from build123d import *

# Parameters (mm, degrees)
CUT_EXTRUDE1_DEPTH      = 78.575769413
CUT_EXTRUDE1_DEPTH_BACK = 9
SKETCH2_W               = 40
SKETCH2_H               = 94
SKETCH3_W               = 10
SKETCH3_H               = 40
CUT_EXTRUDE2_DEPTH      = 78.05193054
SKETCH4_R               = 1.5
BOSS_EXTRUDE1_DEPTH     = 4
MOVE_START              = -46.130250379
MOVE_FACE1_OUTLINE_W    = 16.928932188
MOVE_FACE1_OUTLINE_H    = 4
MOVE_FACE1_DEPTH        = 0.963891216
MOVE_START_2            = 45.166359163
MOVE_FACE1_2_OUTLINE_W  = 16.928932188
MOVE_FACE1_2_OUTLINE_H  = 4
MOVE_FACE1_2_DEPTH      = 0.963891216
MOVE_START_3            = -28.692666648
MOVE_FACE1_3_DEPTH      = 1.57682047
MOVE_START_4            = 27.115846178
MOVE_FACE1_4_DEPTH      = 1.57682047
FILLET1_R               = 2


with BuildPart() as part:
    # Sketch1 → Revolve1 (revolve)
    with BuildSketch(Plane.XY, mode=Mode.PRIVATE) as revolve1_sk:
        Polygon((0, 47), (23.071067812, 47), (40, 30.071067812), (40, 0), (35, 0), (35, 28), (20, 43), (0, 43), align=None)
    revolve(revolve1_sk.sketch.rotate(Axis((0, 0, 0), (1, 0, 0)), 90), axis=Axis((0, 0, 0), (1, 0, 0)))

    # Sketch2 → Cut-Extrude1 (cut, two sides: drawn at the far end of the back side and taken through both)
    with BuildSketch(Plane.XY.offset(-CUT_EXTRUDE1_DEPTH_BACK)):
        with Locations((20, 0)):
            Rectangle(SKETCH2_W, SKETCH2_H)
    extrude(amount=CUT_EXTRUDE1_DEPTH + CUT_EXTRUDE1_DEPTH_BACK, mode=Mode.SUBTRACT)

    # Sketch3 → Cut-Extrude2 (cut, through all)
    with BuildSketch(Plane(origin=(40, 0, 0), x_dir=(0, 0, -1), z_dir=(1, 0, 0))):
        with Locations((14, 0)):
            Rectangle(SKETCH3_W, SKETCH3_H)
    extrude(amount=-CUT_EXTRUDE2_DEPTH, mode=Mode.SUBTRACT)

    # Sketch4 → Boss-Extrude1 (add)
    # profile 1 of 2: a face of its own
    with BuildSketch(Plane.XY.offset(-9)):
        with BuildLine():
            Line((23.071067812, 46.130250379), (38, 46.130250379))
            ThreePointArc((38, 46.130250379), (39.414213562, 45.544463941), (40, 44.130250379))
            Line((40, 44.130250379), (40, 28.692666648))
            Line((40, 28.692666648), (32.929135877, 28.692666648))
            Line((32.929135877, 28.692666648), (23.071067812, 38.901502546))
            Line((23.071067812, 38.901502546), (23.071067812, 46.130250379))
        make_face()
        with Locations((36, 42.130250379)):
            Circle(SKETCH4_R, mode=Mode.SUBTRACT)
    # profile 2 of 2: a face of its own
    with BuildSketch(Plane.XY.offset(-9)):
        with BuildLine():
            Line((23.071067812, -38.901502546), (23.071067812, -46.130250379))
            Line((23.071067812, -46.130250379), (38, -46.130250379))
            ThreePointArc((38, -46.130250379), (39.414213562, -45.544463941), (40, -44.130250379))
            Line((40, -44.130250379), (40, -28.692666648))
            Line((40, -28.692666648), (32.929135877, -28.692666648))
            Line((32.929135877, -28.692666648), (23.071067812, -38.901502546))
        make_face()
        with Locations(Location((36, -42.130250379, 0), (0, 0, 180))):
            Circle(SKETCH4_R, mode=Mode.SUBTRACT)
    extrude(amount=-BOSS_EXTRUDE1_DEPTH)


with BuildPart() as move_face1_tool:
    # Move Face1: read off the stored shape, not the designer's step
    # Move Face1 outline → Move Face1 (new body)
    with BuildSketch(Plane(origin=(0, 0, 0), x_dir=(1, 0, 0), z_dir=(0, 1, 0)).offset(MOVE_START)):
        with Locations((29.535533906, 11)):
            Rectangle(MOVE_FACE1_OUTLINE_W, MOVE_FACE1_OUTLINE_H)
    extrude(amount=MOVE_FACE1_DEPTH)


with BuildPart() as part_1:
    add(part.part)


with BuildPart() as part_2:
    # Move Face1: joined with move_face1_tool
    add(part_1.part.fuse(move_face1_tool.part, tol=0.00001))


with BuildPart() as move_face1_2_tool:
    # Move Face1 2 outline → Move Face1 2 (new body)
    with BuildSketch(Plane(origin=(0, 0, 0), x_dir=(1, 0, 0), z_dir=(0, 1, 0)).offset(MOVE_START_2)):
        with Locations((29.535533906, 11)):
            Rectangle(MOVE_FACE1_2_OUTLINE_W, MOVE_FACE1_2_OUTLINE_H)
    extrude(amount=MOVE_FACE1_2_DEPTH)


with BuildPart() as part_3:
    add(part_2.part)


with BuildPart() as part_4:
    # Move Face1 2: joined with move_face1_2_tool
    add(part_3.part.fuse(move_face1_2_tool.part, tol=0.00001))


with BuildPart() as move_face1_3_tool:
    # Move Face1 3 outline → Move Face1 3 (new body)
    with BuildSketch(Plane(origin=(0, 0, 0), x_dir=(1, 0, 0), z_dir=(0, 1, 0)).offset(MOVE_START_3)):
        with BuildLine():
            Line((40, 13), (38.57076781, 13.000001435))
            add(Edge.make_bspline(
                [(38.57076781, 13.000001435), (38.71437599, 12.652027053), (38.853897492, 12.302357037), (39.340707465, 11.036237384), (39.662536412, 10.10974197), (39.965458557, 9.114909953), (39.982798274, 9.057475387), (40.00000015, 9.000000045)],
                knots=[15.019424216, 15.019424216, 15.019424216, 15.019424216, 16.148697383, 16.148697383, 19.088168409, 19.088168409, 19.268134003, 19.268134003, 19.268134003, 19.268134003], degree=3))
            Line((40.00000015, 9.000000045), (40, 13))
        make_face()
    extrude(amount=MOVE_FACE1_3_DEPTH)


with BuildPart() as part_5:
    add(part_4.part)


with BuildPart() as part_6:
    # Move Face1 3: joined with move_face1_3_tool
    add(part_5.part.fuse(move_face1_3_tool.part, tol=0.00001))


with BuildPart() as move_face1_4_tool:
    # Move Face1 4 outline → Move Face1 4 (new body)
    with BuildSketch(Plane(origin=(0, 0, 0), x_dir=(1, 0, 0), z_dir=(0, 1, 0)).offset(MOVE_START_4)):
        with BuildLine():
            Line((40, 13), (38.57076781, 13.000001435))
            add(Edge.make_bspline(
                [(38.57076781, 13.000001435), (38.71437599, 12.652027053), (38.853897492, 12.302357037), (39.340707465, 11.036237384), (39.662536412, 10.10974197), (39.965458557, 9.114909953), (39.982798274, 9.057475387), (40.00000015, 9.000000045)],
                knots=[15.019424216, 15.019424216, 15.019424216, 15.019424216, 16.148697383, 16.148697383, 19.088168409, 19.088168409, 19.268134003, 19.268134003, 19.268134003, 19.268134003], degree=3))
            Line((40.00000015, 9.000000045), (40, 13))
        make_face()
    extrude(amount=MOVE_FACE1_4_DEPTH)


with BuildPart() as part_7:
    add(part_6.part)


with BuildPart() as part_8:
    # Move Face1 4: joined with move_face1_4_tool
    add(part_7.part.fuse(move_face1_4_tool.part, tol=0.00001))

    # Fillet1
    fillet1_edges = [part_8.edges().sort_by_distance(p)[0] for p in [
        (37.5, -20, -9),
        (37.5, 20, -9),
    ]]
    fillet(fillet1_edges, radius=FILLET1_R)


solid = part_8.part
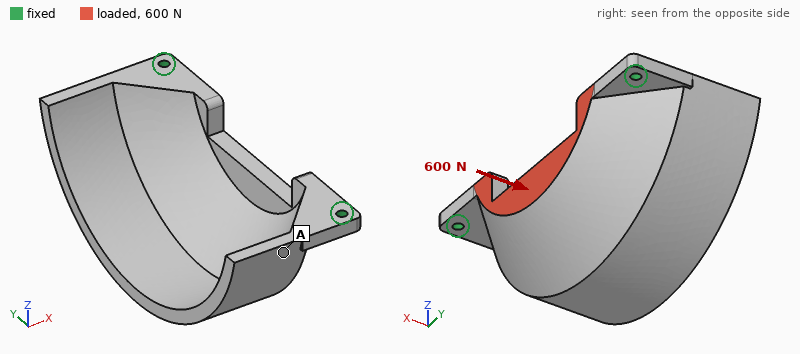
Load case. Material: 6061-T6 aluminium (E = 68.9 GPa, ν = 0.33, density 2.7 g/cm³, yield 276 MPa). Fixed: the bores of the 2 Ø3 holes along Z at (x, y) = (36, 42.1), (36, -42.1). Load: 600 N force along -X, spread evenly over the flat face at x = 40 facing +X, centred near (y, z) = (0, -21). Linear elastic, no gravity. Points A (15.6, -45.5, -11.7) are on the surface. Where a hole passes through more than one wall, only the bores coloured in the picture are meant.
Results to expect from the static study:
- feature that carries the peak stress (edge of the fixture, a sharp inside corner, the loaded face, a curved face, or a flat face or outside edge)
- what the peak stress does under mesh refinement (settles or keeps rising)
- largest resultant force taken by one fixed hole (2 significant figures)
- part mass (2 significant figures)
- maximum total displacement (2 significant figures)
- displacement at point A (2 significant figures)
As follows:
edge of the fixture
keeps rising
340 N
67 g
0.25 mm
0.071 mm
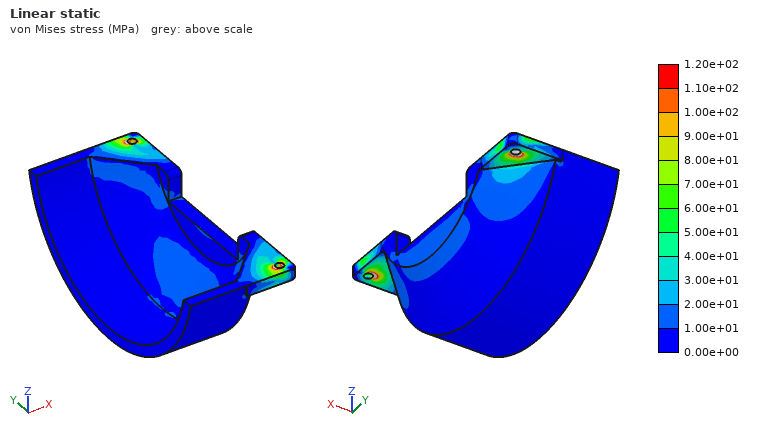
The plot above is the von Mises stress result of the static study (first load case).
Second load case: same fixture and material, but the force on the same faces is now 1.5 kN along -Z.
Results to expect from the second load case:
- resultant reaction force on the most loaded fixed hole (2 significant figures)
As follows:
1.2 kN
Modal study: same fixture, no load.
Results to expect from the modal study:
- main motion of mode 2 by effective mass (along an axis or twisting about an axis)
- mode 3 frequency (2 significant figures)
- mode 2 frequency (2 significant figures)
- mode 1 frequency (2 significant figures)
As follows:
along Y
4300 Hz
2400 Hz
880 Hz
